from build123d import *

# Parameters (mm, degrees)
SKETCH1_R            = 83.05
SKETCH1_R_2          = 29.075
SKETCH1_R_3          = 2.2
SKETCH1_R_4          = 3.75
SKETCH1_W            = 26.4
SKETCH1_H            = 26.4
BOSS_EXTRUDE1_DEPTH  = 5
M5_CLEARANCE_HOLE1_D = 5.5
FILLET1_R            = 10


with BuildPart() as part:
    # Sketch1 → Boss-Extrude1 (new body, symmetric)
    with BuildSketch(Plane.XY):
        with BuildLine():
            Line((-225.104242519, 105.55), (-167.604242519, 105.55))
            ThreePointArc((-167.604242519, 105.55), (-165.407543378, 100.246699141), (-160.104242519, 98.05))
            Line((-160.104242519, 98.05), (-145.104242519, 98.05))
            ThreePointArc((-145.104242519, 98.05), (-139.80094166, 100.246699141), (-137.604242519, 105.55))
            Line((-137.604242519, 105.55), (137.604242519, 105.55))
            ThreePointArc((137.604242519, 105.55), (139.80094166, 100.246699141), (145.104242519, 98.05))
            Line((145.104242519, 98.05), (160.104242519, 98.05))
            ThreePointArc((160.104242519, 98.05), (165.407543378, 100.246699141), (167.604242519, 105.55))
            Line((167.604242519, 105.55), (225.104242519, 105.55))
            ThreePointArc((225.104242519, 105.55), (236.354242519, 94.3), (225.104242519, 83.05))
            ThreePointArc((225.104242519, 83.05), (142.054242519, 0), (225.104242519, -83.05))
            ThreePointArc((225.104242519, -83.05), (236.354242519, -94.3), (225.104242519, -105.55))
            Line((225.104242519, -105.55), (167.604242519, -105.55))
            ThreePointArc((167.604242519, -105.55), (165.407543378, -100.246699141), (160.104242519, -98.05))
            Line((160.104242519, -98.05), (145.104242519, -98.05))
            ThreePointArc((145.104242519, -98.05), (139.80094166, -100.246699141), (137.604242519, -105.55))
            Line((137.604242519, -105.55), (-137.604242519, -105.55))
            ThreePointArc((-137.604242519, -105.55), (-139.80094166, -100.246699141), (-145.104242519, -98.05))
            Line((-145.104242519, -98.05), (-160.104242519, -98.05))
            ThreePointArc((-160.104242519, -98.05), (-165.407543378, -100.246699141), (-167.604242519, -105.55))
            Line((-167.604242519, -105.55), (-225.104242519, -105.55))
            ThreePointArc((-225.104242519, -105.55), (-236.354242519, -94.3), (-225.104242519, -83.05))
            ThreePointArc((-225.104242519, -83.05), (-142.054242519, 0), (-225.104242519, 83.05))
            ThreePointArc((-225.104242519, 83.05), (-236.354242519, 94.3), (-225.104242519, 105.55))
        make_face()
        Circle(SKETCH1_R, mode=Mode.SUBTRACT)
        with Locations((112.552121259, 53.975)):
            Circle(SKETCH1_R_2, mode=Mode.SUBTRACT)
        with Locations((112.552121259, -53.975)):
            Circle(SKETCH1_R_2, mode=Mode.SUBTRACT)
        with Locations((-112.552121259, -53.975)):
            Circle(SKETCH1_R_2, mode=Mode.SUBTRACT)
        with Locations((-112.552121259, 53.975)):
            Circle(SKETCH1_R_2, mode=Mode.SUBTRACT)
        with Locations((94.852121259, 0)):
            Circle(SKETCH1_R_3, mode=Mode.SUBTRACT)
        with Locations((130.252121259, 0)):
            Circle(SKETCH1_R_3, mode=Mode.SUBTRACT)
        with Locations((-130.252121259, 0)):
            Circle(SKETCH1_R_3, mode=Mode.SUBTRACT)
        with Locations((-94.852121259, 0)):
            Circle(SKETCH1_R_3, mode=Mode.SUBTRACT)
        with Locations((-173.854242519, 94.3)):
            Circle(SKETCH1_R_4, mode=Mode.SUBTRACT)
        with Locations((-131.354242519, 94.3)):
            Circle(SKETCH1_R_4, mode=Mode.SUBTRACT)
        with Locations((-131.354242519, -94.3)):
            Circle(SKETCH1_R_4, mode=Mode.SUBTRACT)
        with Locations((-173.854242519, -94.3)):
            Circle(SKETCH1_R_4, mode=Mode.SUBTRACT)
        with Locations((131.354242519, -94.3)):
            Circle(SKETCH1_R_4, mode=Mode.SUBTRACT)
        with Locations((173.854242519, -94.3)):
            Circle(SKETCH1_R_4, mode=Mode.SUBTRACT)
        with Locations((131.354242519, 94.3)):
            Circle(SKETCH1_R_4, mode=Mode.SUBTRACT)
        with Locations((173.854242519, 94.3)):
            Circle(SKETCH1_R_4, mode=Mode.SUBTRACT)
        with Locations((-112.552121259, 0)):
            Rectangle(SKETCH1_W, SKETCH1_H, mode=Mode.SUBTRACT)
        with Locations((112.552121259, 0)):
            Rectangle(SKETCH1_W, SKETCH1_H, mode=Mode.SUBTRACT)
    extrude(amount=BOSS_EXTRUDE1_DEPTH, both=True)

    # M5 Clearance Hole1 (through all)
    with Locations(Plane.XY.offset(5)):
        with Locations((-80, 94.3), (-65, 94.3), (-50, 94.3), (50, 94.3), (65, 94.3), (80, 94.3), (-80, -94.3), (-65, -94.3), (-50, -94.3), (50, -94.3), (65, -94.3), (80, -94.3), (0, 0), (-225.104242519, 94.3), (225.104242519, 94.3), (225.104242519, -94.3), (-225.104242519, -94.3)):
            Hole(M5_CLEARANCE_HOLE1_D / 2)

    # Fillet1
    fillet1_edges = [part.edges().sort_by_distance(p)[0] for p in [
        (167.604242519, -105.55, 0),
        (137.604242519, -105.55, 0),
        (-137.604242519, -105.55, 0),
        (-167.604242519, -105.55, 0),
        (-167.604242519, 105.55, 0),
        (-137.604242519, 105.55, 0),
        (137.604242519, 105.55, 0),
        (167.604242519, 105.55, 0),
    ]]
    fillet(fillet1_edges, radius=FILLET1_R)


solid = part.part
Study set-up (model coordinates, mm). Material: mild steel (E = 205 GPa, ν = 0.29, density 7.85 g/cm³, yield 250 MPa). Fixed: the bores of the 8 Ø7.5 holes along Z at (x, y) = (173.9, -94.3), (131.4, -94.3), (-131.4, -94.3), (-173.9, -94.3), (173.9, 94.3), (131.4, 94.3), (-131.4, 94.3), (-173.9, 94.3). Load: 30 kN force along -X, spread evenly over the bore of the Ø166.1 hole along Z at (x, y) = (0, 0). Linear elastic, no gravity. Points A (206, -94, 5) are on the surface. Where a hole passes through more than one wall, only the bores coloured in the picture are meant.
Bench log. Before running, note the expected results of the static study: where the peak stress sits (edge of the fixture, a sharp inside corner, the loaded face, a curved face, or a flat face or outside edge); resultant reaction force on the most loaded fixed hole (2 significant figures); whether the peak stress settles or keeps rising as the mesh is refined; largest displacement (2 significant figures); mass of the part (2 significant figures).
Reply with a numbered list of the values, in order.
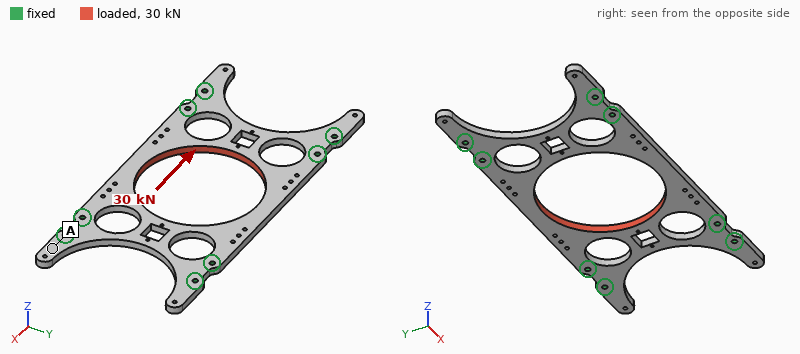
1. edge of the fixture
2. 6.0 kN
3. keeps rising
4. 21 µm
5. 3.0 kg
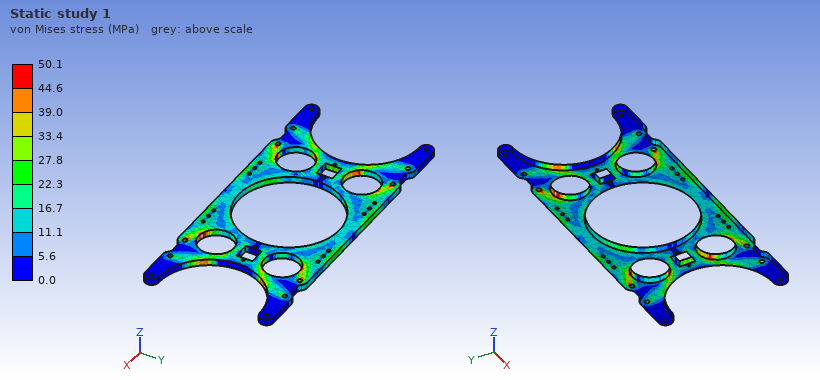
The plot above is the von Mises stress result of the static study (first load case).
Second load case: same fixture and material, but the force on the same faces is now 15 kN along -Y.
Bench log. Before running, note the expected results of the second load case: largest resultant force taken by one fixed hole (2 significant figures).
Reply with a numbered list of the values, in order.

1. 3.4 kN
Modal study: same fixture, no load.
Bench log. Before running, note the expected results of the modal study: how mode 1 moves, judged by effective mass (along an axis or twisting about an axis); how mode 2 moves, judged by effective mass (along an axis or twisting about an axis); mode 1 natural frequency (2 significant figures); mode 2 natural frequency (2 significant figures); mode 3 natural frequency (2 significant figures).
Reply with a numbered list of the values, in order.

1. along Z
2. twisting about X
3. 680 Hz
4. 790 Hz
5. 1200 Hz
